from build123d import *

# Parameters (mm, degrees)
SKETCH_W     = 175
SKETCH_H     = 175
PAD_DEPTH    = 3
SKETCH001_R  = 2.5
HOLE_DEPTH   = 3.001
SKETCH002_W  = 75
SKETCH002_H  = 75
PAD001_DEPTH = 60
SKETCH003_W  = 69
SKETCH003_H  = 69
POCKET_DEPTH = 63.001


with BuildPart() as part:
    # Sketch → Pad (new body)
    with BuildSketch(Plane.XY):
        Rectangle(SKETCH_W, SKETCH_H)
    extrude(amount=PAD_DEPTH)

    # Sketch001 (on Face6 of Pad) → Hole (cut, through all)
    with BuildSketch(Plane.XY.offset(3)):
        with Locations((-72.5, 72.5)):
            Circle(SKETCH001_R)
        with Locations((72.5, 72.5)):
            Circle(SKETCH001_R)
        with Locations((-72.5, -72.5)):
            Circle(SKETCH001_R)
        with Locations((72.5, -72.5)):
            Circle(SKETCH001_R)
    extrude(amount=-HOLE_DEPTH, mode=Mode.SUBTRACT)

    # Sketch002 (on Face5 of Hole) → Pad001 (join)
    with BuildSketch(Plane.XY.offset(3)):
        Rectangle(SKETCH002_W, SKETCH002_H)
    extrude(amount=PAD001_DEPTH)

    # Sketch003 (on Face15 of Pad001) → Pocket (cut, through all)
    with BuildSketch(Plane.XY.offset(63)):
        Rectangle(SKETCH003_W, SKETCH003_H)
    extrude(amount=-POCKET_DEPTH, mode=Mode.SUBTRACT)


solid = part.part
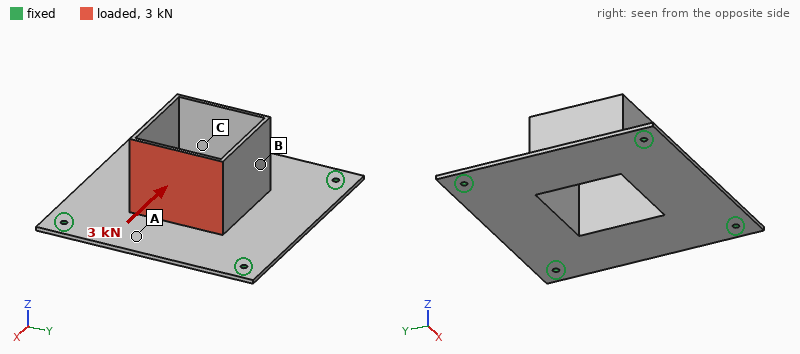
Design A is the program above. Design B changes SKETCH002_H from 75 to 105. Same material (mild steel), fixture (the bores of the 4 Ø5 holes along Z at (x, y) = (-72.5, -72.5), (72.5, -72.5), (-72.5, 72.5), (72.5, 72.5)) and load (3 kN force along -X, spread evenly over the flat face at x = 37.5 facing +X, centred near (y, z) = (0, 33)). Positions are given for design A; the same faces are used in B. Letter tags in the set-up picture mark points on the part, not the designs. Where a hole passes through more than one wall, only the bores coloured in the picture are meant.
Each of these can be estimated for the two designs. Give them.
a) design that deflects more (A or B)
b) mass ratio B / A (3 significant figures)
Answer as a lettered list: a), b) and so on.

a) A
b) 2.04
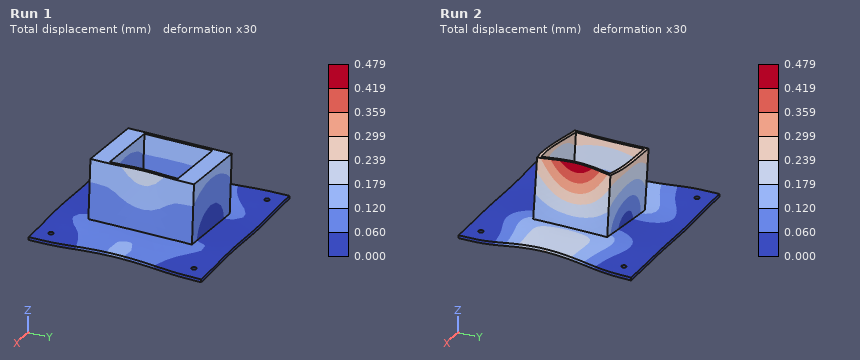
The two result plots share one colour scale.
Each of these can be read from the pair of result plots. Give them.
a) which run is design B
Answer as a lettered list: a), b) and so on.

a) Run 1
